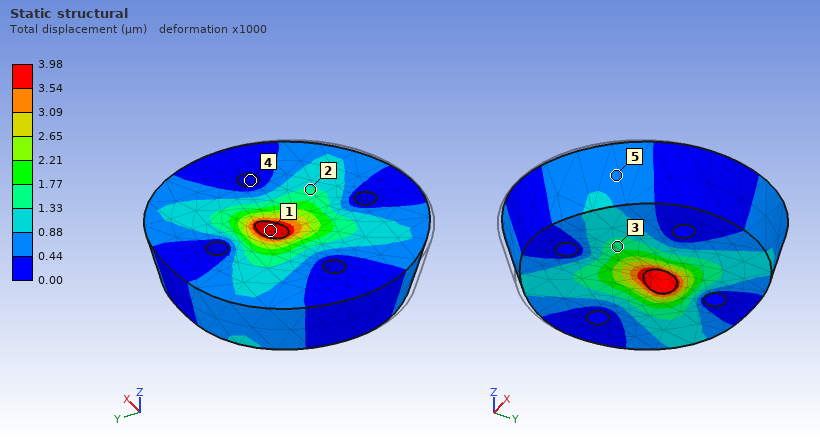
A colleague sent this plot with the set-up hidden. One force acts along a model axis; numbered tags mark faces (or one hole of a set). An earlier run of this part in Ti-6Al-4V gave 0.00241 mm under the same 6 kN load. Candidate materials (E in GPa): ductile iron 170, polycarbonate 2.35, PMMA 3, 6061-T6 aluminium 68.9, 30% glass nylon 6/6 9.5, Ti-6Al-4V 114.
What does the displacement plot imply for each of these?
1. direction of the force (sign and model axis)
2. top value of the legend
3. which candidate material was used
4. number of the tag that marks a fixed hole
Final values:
+Y
3.98 µm
6061-T6 aluminium
4
